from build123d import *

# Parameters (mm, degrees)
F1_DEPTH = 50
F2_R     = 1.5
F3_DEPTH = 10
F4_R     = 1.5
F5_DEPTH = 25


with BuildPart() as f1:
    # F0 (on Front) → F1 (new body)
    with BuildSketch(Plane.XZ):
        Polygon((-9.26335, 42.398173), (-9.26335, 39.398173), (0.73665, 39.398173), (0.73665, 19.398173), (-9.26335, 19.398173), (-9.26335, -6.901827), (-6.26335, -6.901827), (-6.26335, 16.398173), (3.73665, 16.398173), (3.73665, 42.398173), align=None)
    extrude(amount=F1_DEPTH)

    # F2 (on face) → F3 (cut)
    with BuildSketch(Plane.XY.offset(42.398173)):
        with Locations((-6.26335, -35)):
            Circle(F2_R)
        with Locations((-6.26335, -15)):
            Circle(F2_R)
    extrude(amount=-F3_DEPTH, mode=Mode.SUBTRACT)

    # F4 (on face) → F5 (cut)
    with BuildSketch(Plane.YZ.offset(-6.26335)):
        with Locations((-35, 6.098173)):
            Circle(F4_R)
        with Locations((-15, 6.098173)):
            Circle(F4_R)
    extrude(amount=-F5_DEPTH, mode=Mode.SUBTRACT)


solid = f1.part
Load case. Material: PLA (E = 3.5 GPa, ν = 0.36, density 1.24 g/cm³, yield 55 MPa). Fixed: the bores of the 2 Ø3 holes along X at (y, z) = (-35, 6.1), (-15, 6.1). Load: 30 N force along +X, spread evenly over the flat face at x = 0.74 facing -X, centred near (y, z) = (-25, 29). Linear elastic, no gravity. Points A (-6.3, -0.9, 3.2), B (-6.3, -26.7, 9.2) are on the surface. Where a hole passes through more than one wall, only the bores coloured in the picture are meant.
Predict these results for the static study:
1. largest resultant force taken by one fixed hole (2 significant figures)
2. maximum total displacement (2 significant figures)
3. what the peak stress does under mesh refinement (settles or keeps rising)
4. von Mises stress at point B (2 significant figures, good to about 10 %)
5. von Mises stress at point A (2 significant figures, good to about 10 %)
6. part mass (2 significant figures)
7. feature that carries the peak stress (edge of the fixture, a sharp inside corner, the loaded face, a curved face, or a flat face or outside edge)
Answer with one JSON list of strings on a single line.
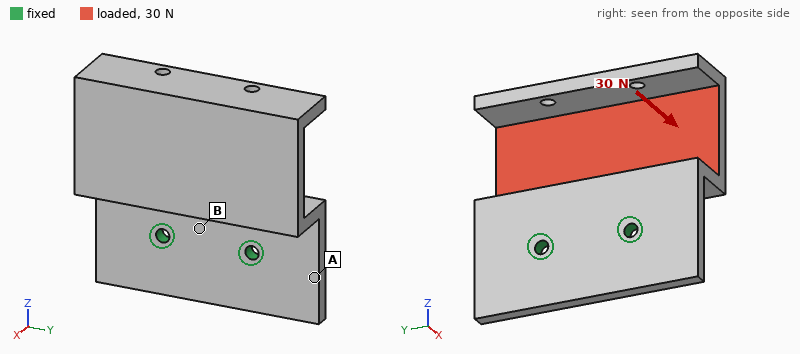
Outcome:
["15 N", "0.85 mm", "keeps rising", "5.9 MPa", "2.2 MPa", "13 g", "edge of the fixture"]
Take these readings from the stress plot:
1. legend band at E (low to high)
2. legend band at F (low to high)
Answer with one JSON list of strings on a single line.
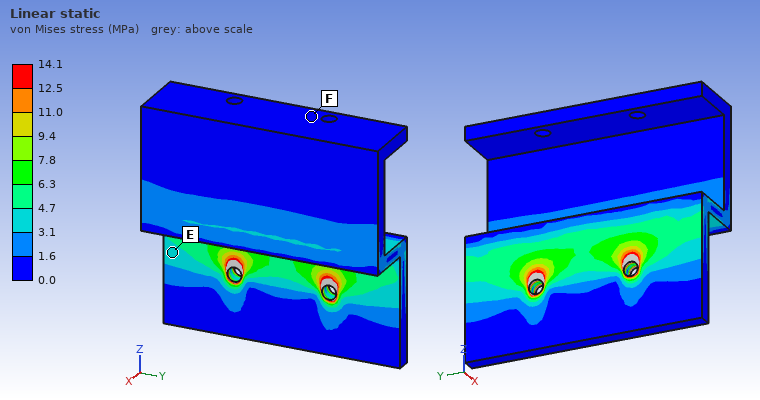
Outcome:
["3.1 to 4.7 MPa", "0.0 to 1.6 MPa"]
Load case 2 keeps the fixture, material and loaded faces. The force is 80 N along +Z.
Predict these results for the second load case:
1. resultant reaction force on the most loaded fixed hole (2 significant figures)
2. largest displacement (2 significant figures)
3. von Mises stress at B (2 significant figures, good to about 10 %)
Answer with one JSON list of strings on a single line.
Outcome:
["40 N", "0.79 mm", "7.2 MPa"]
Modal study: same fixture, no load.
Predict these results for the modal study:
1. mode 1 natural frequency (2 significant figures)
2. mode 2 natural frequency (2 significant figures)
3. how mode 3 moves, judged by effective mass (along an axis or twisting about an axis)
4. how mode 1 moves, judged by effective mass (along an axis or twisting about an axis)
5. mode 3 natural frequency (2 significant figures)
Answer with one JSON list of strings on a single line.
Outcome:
["360 Hz", "780 Hz", "along Z", "along X", "1500 Hz"]
